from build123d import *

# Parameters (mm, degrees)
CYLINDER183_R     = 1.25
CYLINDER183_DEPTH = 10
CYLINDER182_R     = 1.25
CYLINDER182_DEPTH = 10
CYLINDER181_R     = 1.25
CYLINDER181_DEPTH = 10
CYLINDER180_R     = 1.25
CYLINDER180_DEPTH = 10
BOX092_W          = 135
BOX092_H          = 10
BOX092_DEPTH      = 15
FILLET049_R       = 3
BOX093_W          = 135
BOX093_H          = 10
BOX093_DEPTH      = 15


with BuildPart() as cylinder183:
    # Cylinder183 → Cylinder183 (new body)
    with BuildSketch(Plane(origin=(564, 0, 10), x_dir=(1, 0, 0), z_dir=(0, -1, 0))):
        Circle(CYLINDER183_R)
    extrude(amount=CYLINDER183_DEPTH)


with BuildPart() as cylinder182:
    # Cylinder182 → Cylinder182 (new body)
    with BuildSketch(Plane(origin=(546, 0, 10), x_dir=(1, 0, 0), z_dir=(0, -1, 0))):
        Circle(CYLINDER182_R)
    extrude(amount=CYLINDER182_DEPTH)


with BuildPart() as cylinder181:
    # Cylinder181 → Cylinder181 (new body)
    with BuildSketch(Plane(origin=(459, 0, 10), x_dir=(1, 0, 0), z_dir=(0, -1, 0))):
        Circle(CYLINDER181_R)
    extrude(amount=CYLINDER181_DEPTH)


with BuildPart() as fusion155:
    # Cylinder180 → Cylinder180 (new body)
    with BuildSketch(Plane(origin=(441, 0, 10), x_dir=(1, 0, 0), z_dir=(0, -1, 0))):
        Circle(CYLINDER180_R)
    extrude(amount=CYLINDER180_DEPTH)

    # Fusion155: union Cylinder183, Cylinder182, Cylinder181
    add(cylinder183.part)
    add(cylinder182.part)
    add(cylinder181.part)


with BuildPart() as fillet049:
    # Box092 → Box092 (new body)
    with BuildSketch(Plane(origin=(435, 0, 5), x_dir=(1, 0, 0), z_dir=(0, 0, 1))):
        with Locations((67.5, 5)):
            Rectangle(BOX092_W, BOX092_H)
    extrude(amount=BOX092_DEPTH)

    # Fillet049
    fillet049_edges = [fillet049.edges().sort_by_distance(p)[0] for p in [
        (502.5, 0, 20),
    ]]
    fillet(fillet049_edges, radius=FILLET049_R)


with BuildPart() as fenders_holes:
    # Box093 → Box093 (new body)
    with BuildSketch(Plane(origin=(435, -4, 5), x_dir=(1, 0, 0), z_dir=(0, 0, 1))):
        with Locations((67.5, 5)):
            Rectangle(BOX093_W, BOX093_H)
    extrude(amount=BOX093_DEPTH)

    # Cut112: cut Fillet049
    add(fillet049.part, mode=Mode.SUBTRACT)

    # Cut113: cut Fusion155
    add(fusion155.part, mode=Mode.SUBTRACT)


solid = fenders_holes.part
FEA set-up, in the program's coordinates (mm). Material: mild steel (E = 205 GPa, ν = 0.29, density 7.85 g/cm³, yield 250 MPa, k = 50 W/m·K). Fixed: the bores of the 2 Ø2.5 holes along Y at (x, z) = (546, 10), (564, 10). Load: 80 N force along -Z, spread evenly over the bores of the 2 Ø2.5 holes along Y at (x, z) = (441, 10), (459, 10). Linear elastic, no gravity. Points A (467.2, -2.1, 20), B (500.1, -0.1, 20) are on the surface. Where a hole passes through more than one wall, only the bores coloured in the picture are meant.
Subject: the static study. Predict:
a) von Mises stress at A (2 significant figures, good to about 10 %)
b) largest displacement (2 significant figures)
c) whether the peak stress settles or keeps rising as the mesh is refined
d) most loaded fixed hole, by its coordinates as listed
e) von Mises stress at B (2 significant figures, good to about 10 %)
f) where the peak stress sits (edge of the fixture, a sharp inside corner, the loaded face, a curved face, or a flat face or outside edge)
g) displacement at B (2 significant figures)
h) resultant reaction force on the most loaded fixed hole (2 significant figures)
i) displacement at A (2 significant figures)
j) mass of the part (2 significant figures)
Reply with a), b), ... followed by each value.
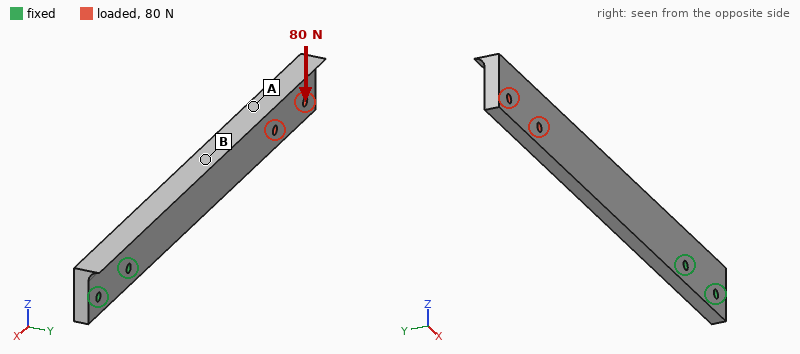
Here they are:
a) 8.4 MPa
b) 0.15 mm
c) keeps rising
d) (546, 10)
e) 22 MPa
f) edge of the fixture
g) 0.041 mm
h) 500 N
i) 0.094 mm
j) 65 g
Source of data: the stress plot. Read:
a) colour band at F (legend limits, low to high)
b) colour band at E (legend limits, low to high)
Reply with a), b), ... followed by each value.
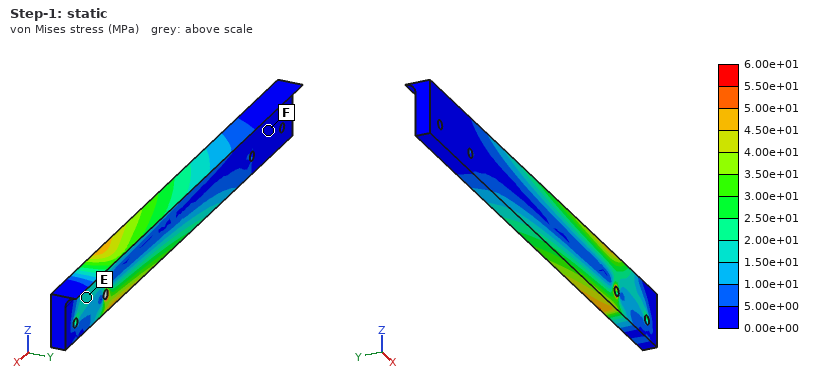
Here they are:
a) 0.00e+00 to 5.00e+00 MPa
b) 1.50e+01 to 2.00e+01 MPa
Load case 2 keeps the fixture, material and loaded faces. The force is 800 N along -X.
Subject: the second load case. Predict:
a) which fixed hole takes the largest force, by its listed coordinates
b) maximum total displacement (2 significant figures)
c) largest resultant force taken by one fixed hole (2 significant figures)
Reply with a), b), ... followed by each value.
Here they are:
a) (546, 10)
b) 54 µm
c) 710 N
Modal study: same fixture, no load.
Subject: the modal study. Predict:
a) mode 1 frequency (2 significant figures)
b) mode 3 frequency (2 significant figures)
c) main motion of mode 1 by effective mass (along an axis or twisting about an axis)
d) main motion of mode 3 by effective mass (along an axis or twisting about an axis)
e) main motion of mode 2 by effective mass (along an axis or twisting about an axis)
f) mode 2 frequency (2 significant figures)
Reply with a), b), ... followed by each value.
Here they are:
a) 280 Hz
b) 1700 Hz
c) along Y
d) along Y
e) along Z
f) 910 Hz
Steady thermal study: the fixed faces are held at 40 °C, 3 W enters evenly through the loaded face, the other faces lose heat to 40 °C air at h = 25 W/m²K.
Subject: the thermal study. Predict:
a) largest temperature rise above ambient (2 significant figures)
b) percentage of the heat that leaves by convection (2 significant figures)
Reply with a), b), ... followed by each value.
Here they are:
a) 40 K
b) 75 %
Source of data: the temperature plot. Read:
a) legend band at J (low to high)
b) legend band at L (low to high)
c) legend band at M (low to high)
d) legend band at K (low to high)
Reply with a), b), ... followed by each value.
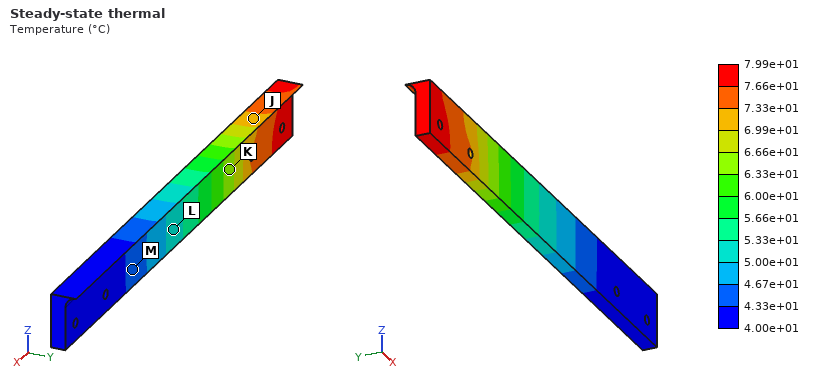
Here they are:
a) 6.99e+01 to 7.33e+01 °C
b) 5.00e+01 to 5.33e+01 °C
c) 4.33e+01 to 4.67e+01 °C
d) 6.33e+01 to 6.66e+01 °C
